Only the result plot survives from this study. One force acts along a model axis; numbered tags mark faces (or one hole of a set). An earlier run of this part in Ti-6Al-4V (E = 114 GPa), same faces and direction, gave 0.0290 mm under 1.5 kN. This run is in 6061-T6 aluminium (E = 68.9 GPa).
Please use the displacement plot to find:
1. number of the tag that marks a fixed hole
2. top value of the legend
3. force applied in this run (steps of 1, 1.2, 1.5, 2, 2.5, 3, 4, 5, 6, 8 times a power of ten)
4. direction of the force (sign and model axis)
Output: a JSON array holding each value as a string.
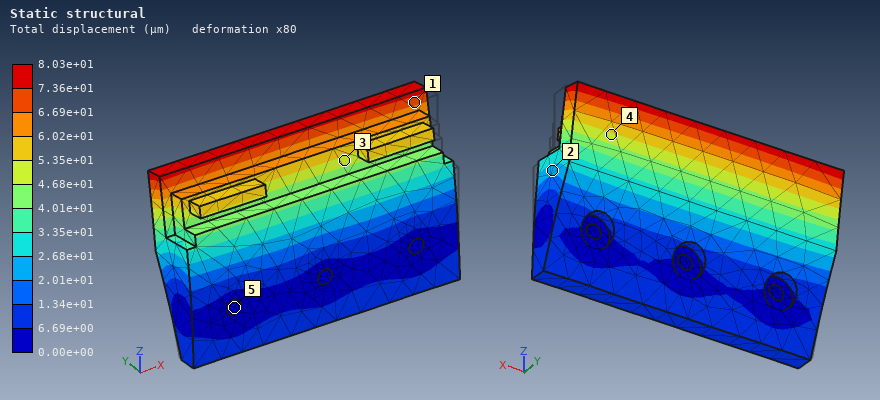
["5", "8.03e+01 µm", "2.5 kN", "+Y"]
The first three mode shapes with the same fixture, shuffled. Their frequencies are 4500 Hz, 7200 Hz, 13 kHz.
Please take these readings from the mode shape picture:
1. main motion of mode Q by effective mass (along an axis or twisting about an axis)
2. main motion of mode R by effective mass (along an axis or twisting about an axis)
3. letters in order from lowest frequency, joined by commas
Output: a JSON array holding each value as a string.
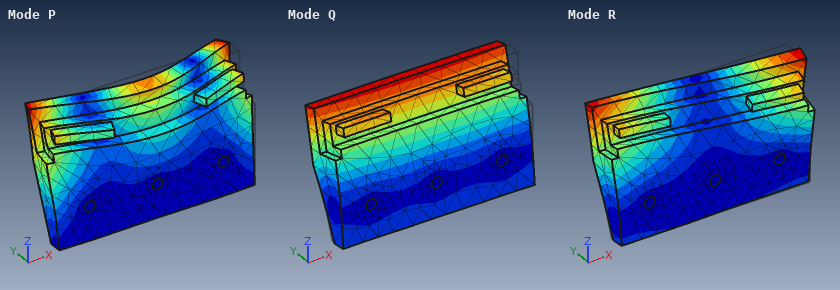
["along Y", "twisting about Z", "Q, R, P"]
